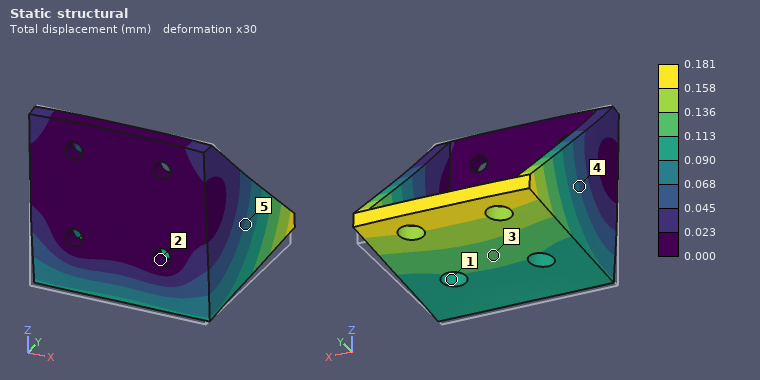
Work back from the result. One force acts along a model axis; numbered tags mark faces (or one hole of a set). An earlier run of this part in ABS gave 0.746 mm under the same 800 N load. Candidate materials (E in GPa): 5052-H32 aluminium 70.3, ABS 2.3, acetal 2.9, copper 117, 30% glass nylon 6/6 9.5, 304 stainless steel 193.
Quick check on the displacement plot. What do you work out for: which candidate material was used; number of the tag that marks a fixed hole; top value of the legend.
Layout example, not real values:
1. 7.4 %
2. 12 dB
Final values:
1. 30% glass nylon 6/6
2. 2
3. 0.181 mm
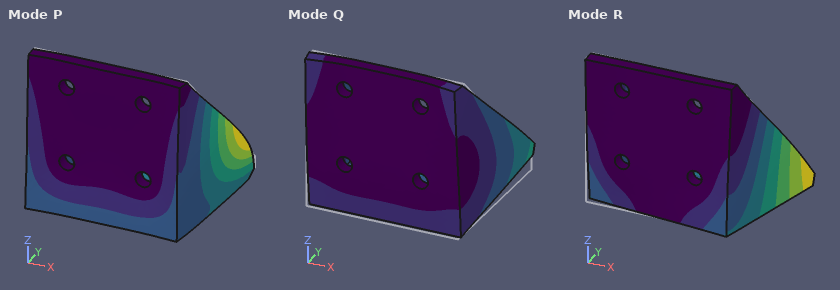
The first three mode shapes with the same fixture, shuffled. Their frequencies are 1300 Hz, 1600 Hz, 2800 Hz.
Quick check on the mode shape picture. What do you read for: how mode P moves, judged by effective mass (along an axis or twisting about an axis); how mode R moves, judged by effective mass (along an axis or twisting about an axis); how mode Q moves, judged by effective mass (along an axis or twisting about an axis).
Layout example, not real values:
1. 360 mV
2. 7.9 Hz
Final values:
1. along Y
2. along X
3. along Z
